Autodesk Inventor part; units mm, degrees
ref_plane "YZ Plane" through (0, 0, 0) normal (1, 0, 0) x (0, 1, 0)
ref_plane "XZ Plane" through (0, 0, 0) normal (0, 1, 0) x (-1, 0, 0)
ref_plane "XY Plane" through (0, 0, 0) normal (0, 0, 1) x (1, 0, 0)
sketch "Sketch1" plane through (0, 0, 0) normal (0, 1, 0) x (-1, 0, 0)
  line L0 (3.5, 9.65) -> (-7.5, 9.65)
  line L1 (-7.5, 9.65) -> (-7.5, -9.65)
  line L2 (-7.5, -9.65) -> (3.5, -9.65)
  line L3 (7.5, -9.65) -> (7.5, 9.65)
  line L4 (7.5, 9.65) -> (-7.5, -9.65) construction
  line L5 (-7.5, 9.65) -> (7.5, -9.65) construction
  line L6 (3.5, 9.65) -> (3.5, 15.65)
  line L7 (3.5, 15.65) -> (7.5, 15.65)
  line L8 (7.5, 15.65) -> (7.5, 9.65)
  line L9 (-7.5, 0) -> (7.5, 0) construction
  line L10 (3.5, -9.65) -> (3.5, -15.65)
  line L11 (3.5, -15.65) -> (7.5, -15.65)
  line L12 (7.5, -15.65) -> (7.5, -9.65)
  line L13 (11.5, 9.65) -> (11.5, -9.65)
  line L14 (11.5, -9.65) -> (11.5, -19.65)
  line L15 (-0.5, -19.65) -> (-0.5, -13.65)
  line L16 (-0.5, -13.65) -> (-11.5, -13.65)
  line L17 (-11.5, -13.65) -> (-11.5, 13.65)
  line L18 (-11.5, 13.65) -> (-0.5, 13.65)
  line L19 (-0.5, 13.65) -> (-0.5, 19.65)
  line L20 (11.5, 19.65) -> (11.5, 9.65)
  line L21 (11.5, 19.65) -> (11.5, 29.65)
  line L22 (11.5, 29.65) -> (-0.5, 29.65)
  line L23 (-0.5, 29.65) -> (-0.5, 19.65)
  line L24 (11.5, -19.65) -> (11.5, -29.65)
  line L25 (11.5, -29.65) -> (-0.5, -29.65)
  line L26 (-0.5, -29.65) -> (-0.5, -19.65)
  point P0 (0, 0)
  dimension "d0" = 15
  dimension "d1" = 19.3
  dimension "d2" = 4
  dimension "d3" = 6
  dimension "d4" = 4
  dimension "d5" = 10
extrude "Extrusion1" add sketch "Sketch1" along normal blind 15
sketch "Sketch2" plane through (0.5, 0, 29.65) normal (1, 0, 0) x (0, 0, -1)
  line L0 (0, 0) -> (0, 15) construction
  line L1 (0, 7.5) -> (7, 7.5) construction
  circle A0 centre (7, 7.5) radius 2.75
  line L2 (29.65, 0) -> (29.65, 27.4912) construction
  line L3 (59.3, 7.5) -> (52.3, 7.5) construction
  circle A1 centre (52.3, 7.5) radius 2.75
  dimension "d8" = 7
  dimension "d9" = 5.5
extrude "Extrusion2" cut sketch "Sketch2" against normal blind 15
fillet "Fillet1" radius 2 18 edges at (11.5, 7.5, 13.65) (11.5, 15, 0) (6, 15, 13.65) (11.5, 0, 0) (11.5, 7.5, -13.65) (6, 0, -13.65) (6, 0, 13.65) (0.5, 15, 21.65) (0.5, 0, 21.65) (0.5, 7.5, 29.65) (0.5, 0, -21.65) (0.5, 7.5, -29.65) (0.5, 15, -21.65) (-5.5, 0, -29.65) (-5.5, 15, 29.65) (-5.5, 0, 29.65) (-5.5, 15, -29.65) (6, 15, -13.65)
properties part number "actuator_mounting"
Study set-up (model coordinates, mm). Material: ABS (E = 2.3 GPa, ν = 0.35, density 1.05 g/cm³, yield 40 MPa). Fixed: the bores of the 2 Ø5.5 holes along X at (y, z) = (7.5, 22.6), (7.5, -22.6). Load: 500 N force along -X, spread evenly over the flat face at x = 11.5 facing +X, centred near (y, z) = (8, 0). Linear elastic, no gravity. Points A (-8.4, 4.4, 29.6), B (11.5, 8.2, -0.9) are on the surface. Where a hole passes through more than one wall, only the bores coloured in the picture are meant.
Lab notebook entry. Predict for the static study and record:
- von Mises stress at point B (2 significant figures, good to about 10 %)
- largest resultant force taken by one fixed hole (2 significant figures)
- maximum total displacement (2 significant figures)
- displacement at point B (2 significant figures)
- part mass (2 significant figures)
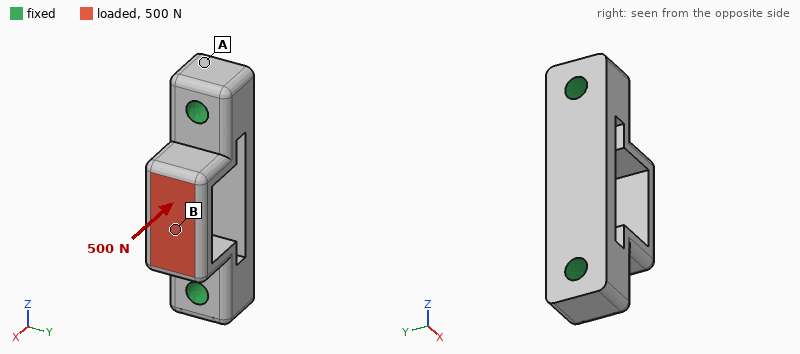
14 MPa
280 N
0.21 mm
0.20 mm
9.8 g
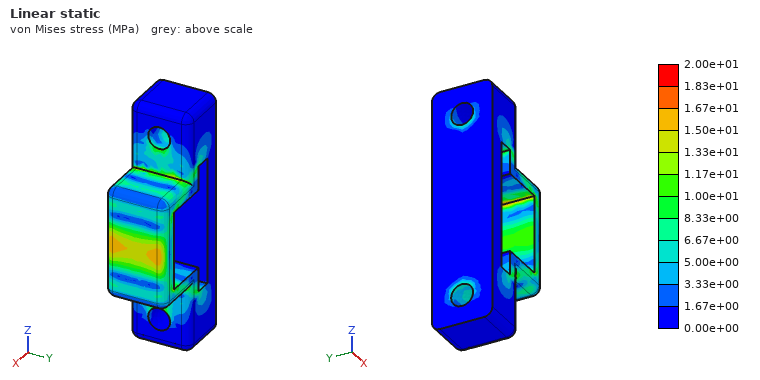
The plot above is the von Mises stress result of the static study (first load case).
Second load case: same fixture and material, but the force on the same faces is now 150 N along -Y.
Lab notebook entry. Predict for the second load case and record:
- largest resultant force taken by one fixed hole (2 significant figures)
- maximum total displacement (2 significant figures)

75 N
0.22 mm
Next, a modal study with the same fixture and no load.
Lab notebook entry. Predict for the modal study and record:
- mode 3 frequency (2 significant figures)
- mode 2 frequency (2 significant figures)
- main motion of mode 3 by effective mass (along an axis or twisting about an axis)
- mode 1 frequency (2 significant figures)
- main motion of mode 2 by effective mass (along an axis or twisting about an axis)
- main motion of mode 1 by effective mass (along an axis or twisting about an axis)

4500 Hz
3900 Hz
along X
3400 Hz
along Z
along Y
